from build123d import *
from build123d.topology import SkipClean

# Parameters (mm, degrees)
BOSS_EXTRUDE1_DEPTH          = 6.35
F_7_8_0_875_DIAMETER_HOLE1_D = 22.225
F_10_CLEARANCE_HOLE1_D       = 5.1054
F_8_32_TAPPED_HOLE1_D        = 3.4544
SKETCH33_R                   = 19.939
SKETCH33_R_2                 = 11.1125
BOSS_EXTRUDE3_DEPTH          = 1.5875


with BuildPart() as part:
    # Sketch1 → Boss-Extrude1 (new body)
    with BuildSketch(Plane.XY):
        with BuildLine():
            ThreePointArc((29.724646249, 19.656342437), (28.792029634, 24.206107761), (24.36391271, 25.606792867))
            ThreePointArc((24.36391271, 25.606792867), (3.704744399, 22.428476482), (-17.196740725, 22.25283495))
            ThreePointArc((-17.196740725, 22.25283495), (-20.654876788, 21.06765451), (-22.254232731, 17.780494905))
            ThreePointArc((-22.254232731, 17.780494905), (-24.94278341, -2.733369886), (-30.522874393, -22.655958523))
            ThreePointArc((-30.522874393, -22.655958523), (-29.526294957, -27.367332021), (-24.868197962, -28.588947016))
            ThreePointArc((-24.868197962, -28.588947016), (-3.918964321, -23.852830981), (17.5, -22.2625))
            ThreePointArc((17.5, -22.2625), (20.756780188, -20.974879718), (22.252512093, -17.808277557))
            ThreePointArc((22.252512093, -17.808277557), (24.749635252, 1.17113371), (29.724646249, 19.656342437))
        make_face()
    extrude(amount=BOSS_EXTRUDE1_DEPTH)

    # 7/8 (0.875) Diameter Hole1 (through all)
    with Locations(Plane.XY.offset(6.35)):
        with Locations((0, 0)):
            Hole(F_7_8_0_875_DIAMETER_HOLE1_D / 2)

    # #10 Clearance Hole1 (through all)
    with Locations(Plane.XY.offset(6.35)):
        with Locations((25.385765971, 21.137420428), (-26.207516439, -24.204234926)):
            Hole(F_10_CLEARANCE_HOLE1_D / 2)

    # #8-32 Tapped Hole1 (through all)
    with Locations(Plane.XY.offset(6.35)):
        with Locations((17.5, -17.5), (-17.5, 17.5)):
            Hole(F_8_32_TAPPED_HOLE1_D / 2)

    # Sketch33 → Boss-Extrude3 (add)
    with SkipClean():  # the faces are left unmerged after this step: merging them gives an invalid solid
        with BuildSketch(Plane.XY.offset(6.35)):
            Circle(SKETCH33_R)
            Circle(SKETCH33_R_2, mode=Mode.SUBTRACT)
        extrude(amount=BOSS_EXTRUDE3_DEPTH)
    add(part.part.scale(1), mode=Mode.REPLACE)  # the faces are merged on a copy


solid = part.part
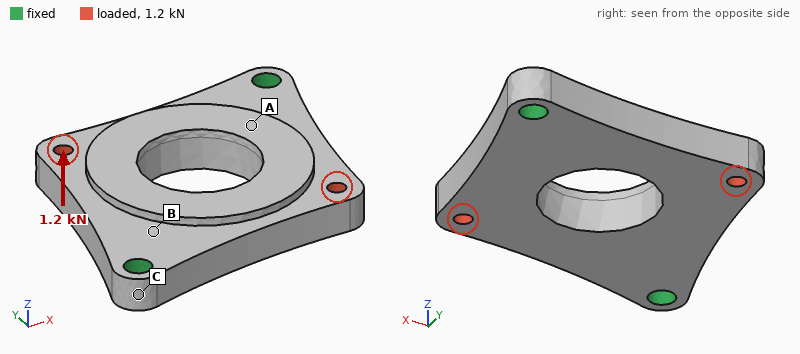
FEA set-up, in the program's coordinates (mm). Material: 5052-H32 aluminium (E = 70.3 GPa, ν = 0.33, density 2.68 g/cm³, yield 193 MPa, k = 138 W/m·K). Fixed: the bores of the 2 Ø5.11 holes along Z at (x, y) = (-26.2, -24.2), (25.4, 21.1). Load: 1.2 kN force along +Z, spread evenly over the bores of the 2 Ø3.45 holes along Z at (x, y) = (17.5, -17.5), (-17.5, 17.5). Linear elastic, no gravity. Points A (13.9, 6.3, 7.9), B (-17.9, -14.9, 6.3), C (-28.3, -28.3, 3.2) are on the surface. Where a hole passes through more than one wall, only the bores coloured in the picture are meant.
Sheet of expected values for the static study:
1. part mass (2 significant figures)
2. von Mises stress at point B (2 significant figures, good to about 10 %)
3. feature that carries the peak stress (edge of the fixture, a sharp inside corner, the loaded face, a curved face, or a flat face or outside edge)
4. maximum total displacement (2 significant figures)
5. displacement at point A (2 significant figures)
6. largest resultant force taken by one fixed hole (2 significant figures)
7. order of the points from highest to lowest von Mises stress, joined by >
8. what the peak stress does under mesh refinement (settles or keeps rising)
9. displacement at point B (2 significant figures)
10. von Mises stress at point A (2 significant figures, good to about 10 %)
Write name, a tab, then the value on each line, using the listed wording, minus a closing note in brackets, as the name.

part mass	37 g
von Mises stress at point B	23 MPa
feature that carries the peak stress	edge of the fixture
maximum total displacement	0.13 mm
displacement at point A	0.034 mm
largest resultant force taken by one fixed hole	730 N
order of the points from highest to lowest von Mises stress, joined by >	A > B > C
what the peak stress does under mesh refinement	keeps rising
displacement at point B	0.020 mm
von Mises stress at point A	44 MPa
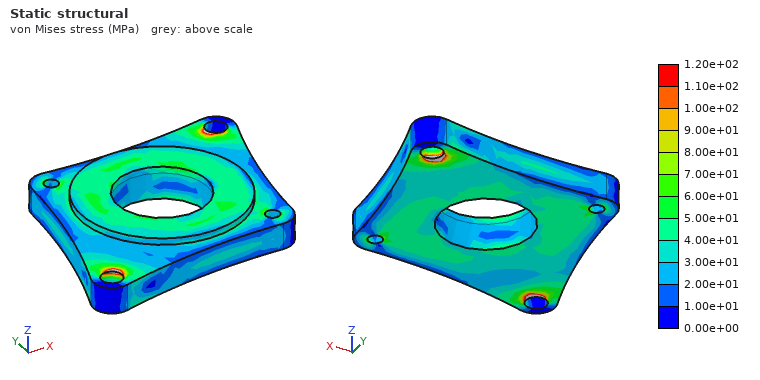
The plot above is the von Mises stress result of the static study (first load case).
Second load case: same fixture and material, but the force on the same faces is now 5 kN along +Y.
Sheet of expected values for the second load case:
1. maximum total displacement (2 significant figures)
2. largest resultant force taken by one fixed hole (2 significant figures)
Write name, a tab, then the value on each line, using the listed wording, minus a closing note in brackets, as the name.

maximum total displacement	27 µm
largest resultant force taken by one fixed hole	2.5 kN
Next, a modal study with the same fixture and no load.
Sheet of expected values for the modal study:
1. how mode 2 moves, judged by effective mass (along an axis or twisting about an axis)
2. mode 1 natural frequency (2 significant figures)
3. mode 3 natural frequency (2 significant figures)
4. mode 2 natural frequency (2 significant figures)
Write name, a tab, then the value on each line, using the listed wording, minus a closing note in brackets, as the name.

how mode 2 moves, judged by effective mass	along Z
mode 1 natural frequency	4100 Hz
mode 3 natural frequency	13 kHz
mode 2 natural frequency	5000 Hz
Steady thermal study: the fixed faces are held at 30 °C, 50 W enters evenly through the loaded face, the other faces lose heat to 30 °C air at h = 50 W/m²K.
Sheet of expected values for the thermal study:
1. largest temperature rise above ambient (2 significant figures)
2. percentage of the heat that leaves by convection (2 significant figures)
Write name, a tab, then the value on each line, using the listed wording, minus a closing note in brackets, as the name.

largest temperature rise above ambient	54 K
percentage of the heat that leaves by convection	15 %
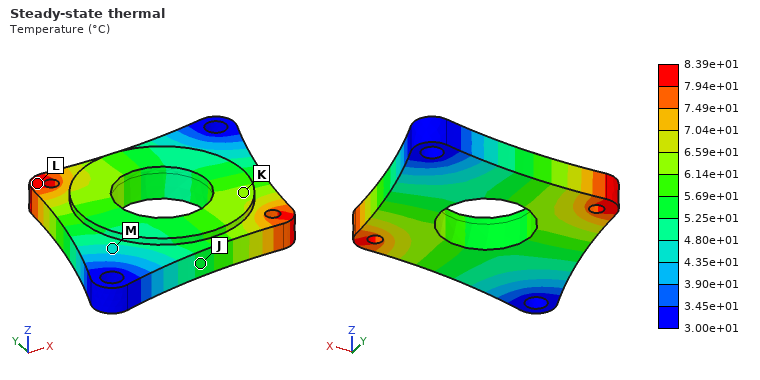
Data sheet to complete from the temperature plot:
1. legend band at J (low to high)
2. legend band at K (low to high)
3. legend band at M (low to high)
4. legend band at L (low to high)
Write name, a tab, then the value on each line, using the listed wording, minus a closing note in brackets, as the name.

legend band at J	5.25e+01 to 5.69e+01 °C
legend band at K	6.14e+01 to 6.59e+01 °C
legend band at M	4.35e+01 to 4.80e+01 °C
legend band at L	7.94e+01 to 8.39e+01 °C
